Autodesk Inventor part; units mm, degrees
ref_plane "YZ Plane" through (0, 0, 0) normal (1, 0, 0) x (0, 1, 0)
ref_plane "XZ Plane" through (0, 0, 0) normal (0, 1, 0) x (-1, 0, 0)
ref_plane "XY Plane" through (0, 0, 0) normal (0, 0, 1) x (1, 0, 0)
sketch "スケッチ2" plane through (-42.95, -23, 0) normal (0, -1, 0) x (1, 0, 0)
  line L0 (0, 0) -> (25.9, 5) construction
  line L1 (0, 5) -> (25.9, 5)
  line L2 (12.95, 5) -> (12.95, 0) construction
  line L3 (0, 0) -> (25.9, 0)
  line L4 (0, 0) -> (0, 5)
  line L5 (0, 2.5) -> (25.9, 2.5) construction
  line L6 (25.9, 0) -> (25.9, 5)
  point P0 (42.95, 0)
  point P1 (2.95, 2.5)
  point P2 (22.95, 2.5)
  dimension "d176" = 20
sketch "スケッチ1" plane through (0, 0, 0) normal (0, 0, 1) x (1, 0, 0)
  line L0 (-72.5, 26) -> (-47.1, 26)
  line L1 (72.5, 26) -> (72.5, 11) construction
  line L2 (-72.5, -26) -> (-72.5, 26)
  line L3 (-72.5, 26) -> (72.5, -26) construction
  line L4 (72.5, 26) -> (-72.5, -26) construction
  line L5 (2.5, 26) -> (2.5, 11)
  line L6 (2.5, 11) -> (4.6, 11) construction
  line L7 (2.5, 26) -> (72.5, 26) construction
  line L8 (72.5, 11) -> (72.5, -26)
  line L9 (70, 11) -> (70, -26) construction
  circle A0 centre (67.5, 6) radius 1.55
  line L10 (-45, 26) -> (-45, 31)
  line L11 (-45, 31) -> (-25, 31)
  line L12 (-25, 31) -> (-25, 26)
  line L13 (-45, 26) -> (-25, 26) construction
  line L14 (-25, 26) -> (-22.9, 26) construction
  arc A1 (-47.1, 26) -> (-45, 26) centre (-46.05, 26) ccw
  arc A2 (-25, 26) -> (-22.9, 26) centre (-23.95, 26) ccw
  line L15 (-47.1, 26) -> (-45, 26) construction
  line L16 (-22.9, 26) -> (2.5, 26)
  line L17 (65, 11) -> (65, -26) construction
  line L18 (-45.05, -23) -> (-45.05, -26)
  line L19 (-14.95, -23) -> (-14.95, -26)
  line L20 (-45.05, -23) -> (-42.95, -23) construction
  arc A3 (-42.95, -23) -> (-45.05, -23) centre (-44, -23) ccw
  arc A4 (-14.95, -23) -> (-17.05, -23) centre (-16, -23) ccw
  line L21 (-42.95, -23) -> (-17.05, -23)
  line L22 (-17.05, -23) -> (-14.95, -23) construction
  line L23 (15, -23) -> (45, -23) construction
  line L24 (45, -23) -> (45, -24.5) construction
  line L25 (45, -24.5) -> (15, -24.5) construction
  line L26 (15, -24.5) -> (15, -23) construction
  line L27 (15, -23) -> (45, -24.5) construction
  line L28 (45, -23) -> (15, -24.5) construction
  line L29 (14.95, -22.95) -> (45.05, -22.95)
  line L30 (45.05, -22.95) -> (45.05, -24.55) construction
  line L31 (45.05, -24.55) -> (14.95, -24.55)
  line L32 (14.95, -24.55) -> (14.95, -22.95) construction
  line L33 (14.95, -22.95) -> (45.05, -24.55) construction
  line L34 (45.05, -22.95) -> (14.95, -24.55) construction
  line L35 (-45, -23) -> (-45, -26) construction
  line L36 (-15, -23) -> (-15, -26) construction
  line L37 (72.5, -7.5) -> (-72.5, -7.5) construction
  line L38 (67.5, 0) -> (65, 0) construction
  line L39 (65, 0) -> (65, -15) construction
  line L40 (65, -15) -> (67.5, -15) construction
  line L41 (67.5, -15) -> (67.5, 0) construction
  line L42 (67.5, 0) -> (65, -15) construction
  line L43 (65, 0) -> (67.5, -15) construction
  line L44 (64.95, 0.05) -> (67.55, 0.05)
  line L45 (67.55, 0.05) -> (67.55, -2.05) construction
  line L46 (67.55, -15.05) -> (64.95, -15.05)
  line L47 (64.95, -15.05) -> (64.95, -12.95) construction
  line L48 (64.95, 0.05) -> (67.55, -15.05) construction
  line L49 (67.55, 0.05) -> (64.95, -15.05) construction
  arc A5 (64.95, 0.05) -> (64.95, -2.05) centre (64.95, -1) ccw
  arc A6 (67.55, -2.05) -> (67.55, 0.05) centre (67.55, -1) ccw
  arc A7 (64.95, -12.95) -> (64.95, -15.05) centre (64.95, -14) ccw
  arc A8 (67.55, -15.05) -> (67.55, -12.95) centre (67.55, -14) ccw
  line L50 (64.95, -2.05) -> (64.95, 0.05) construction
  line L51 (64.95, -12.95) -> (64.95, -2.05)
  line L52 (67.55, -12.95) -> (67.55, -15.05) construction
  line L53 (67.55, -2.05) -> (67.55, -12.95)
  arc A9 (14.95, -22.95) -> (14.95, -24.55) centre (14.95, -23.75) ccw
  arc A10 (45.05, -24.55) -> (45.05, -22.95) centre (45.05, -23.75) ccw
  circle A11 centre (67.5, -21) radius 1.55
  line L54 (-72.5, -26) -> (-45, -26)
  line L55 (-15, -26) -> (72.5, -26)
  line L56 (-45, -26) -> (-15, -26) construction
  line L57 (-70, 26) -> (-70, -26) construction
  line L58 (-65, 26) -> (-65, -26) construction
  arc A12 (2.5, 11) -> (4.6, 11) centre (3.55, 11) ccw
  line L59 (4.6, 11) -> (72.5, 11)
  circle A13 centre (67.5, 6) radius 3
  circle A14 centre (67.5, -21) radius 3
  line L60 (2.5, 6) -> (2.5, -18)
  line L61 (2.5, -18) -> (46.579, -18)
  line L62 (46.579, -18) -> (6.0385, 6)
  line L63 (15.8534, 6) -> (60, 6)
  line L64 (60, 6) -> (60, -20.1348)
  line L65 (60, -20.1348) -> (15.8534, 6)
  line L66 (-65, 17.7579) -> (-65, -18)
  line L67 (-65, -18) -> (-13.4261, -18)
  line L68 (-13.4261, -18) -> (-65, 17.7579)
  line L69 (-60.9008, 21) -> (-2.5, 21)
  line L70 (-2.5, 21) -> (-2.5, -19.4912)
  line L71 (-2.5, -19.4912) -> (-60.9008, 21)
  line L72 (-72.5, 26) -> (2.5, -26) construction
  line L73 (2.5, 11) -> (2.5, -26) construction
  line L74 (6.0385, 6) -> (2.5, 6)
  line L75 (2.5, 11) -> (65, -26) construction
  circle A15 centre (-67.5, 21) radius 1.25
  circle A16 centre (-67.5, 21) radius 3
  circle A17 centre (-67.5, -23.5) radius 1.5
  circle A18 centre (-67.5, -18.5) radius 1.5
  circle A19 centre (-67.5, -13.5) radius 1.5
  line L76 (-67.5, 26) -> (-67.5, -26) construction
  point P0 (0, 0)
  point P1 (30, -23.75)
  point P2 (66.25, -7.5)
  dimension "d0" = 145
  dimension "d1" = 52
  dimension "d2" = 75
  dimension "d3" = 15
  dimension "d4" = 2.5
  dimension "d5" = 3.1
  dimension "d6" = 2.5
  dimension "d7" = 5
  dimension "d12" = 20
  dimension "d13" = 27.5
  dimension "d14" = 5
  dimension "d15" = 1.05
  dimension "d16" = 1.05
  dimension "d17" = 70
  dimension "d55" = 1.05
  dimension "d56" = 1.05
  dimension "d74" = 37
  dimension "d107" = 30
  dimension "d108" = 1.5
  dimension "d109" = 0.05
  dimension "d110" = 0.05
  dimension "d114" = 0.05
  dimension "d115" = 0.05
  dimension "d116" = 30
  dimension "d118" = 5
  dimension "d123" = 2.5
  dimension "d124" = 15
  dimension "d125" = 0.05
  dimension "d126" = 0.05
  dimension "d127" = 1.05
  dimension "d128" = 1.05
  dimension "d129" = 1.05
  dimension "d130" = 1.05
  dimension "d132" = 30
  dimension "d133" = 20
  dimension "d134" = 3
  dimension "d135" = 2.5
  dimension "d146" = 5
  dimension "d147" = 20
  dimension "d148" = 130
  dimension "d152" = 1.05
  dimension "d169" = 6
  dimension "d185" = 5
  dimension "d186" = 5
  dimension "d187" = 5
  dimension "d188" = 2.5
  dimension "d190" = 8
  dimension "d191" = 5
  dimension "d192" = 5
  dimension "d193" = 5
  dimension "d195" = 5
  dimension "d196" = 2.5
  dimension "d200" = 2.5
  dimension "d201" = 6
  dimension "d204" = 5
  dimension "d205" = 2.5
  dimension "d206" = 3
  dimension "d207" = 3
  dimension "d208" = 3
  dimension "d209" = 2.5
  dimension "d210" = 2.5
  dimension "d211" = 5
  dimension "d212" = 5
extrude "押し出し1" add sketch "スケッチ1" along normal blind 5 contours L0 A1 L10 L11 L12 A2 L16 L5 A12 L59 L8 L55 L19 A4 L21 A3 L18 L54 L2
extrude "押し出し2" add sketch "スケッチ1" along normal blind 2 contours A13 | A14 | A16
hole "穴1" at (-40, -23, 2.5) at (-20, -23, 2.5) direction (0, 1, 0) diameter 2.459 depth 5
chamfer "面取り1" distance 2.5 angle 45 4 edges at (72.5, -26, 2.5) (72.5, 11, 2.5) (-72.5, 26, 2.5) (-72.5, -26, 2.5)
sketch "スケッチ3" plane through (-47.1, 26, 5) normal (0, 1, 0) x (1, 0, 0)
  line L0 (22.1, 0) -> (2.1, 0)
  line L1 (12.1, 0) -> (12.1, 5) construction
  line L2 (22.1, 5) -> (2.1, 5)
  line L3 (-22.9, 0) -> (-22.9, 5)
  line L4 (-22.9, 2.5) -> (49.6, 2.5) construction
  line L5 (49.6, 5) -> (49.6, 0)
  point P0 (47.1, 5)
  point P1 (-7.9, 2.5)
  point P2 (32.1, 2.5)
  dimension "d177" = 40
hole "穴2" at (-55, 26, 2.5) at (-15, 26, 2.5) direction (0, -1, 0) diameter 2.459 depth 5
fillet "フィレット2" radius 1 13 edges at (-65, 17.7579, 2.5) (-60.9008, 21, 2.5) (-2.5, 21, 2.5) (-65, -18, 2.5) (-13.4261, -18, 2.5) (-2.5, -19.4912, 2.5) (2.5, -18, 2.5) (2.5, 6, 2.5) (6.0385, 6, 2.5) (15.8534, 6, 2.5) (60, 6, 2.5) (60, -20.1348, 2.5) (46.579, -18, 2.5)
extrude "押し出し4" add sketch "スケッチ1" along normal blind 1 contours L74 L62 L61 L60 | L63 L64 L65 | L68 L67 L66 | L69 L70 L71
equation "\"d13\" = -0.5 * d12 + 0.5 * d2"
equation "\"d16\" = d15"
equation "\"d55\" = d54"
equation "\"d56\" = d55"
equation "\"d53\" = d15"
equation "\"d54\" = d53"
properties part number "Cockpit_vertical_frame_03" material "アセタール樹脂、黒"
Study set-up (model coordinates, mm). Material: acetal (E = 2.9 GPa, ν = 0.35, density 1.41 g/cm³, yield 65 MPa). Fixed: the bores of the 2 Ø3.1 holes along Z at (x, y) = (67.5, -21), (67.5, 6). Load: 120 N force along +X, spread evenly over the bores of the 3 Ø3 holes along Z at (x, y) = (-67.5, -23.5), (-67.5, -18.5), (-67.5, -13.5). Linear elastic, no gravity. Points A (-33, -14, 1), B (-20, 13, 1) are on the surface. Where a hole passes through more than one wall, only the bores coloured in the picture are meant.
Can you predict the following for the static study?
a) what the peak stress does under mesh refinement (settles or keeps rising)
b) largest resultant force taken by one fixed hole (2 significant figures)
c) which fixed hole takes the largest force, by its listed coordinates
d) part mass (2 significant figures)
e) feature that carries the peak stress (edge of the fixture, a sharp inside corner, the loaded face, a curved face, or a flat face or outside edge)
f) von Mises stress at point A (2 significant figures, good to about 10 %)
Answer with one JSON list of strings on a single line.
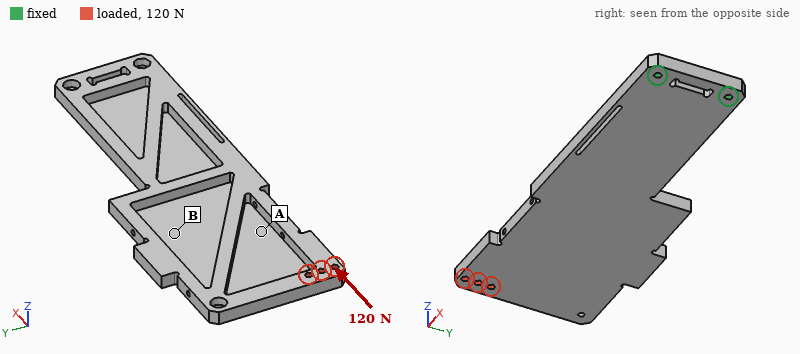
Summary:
["keeps rising", "110 N", "(67.5, -21)", "26 g", "edge of the fixture", "2.6 MPa"]
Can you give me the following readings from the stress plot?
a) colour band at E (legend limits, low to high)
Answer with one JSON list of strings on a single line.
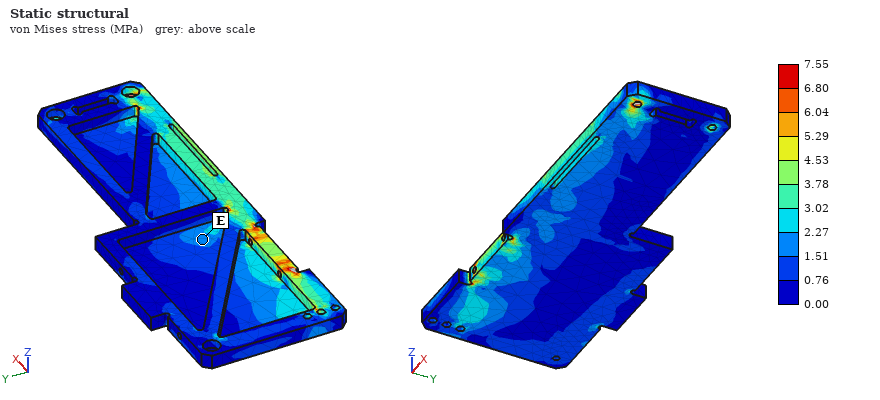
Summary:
["1.51 to 2.27 MPa"]
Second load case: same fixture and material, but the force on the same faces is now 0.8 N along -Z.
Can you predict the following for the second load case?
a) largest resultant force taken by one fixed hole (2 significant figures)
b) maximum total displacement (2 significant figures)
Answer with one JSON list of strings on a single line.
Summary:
["3.1 N", "1.5 mm"]
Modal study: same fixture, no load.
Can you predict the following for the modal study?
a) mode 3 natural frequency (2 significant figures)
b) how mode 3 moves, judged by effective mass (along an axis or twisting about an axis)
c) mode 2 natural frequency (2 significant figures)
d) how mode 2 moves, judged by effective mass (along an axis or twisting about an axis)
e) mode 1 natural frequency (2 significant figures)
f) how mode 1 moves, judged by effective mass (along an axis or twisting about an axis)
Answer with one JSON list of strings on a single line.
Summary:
["270 Hz", "along Z", "180 Hz", "twisting about X", "43 Hz", "along Z"]
